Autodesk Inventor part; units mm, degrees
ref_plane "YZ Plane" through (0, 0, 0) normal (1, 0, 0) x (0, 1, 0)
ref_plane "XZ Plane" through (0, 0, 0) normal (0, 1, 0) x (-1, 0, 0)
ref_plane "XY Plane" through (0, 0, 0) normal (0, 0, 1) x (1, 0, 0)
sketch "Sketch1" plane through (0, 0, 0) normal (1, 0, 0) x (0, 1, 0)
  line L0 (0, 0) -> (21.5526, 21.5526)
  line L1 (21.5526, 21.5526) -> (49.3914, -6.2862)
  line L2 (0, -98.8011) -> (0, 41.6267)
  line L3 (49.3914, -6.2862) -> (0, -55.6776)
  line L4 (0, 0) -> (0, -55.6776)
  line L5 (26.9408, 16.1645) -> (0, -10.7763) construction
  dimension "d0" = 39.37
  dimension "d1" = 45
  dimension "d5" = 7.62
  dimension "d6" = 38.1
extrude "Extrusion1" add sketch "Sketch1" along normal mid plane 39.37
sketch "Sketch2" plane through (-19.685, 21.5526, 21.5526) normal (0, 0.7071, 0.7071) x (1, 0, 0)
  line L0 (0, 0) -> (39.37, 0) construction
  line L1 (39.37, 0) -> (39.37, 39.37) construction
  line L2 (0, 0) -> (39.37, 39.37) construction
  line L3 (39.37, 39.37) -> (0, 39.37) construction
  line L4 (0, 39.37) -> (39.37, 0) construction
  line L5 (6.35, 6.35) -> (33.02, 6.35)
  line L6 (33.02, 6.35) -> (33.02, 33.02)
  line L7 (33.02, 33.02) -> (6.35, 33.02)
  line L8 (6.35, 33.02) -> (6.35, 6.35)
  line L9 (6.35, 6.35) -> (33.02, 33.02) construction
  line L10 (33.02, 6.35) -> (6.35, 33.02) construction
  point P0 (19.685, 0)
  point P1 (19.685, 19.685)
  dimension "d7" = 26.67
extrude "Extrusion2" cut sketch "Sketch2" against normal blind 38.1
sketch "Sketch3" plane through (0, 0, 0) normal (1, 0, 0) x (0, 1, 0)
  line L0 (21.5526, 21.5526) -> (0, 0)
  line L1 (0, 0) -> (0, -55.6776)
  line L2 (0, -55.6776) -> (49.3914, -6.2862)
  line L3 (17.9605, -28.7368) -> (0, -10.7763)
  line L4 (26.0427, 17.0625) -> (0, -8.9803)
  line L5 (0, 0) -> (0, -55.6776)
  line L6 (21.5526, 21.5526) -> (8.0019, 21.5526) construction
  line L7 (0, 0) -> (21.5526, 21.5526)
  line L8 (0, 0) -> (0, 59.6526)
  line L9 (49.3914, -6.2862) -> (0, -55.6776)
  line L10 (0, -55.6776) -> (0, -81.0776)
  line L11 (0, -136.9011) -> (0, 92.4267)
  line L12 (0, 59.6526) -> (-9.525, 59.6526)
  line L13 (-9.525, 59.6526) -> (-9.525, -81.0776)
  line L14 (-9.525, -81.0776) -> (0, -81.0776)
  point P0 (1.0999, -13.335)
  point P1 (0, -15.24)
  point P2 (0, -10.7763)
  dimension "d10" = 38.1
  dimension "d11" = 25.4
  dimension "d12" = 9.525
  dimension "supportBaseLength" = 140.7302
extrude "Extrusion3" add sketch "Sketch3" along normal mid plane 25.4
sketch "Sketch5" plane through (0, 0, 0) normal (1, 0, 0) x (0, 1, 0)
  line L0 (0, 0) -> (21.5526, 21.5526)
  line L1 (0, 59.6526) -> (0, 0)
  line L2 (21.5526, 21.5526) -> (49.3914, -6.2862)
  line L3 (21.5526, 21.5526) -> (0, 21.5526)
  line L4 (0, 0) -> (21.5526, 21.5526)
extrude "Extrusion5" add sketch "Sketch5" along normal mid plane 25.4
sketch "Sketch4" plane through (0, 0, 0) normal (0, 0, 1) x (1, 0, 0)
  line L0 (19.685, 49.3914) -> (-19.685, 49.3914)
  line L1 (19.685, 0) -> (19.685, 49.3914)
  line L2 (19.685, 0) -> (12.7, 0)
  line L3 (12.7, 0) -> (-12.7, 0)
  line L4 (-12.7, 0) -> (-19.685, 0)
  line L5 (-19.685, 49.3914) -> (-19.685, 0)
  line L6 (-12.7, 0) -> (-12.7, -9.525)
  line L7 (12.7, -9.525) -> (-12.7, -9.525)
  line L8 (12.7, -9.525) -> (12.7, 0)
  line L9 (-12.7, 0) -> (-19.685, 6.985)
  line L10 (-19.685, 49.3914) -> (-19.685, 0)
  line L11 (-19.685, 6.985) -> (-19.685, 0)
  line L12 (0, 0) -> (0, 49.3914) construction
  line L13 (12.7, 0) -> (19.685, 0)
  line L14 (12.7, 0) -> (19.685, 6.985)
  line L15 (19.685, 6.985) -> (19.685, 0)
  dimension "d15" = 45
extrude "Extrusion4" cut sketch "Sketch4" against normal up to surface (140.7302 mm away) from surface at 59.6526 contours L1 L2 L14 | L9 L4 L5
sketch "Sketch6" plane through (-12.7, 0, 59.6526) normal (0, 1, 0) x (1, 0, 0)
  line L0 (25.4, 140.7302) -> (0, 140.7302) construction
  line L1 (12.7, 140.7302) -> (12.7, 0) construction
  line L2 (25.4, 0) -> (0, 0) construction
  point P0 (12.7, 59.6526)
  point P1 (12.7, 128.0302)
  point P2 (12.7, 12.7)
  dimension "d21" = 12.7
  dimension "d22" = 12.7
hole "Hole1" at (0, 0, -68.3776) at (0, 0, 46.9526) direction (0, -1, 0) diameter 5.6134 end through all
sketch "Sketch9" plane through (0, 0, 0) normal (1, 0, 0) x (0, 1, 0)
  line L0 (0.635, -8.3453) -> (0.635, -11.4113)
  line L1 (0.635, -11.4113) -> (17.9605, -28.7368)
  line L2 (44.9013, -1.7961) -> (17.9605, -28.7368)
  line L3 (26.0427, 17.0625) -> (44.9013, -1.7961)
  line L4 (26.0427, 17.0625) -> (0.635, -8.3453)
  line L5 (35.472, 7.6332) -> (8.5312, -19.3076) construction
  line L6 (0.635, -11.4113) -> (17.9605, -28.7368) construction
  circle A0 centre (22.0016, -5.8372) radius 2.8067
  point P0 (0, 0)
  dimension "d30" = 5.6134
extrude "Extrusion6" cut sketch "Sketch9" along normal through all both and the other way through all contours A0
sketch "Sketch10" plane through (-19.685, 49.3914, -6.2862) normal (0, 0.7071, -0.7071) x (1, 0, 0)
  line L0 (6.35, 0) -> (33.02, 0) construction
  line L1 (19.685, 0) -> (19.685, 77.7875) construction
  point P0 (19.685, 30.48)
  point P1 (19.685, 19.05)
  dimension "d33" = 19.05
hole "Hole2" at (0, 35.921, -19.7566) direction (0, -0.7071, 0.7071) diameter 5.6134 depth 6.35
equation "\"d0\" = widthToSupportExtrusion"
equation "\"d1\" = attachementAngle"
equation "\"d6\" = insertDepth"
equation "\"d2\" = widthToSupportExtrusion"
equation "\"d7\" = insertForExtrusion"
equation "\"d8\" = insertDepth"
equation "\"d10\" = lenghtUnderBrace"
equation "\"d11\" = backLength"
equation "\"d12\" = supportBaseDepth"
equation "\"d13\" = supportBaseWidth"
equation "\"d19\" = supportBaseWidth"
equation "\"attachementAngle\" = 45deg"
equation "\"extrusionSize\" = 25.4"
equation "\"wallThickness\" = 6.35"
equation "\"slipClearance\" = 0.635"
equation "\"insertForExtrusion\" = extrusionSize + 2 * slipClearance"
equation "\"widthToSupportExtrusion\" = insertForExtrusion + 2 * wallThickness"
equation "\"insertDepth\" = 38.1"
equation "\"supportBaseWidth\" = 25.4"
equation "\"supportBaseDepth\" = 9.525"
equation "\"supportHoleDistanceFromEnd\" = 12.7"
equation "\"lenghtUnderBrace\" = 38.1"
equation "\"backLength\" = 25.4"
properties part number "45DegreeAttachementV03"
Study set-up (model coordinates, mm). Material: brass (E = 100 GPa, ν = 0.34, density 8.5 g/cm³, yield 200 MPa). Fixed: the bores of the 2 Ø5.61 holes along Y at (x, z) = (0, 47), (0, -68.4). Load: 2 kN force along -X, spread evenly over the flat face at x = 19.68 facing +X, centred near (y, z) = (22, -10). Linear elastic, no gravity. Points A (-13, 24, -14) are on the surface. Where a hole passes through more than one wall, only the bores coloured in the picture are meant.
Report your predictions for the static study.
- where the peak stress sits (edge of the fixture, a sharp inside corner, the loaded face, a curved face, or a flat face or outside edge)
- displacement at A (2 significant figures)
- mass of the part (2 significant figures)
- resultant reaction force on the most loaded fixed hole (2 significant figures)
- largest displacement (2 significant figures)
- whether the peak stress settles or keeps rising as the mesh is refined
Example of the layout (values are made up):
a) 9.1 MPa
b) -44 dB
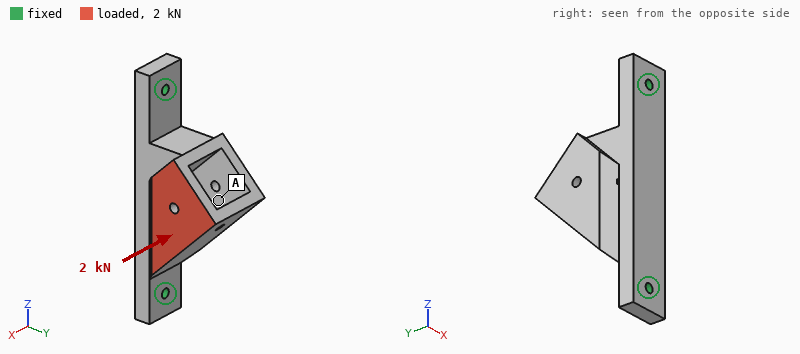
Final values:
a) edge of the fixture
b) 0.097 mm
c) 740 g
d) 1.0 kN
e) 0.17 mm
f) keeps rising
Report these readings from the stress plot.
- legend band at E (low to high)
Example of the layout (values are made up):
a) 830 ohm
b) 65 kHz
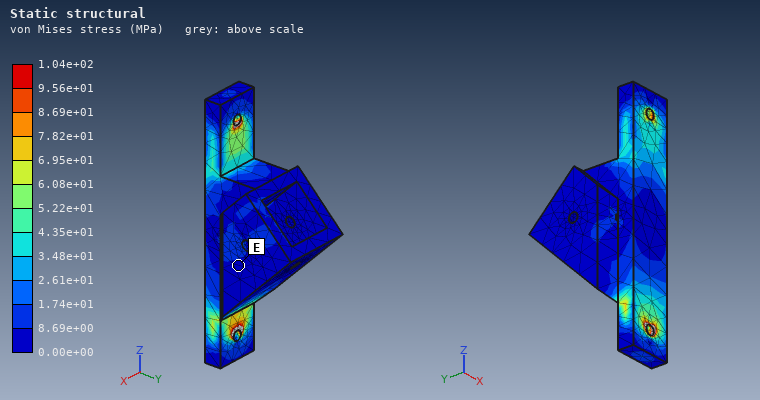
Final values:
a) 0.00e+00 to 8.69e+00 MPa
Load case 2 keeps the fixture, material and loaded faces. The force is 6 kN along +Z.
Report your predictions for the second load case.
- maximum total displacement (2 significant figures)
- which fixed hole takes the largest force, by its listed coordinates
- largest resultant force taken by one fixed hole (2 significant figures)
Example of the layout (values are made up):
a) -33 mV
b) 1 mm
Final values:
a) 42 µm
b) (0, -68.4)
c) 4.0 kN
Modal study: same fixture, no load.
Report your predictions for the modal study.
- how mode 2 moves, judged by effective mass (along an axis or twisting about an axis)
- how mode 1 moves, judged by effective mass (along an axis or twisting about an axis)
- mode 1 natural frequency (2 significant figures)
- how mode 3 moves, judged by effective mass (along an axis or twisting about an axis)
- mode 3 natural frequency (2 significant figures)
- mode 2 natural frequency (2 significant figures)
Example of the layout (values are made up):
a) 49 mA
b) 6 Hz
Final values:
a) along Y
b) along X
c) 1200 Hz
d) along X
e) 3700 Hz
f) 2300 Hz
